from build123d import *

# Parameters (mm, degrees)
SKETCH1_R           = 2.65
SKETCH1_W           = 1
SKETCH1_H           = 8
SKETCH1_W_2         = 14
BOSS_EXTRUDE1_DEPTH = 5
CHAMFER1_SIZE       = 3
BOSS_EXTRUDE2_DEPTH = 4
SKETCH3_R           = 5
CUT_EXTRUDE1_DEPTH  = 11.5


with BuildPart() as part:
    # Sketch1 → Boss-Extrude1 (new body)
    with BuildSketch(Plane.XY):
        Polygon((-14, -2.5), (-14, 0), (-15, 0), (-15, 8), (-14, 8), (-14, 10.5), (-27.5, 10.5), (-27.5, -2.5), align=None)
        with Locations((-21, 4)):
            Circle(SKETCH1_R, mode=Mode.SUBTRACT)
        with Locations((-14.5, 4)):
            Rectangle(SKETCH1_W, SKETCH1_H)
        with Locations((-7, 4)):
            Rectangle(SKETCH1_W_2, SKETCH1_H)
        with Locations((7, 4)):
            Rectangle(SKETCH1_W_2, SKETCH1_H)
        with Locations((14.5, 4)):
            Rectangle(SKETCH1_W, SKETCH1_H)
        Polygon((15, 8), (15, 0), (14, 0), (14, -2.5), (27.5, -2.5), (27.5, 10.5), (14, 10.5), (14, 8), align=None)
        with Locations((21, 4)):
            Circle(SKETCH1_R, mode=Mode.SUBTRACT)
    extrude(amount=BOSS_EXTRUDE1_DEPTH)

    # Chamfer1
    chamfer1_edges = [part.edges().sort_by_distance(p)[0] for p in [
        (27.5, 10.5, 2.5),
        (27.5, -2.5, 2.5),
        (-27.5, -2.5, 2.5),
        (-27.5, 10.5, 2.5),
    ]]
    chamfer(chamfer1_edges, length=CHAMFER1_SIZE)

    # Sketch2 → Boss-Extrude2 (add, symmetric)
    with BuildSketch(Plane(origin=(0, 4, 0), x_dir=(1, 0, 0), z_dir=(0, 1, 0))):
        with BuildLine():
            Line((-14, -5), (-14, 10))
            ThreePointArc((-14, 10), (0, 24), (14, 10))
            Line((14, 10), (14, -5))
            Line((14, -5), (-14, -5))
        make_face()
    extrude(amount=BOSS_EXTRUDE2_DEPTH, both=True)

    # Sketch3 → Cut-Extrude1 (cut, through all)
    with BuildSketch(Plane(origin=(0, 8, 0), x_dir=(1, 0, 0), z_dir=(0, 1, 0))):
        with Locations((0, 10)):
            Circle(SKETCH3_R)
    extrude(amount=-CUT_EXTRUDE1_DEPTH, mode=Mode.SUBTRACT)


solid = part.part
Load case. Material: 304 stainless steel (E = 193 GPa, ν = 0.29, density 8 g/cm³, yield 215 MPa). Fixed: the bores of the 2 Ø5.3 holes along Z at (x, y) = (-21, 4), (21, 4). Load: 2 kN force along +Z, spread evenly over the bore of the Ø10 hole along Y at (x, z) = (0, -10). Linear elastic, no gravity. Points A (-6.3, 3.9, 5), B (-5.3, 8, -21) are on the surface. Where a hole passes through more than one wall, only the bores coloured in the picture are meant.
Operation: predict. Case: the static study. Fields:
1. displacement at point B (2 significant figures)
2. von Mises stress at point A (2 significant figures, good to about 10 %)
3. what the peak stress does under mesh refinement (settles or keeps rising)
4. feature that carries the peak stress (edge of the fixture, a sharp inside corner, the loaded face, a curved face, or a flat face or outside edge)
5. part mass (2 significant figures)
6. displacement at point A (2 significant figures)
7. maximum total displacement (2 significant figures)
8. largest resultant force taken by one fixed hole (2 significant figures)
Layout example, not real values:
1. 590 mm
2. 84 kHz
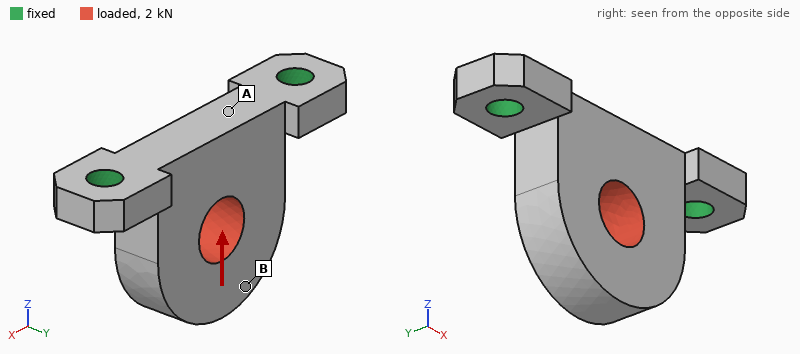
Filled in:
1. 5.5 µm
2. 18 MPa
3. keeps rising
4. edge of the fixture
5. 53 g
6. 5.4 µm
7. 6.1 µm
8. 1.1 kN
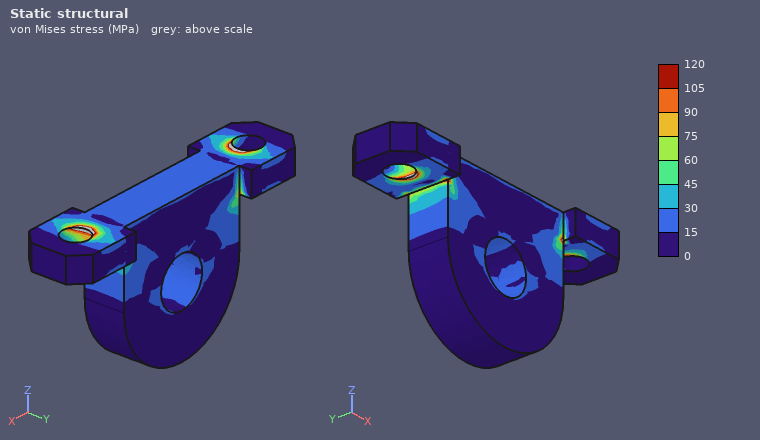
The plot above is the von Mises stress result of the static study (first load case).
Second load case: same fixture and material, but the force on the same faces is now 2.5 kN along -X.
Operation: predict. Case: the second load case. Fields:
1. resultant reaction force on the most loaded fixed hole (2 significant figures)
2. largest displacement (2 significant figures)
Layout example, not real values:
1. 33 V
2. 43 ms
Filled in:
1. 1.6 kN
2. 11 µm
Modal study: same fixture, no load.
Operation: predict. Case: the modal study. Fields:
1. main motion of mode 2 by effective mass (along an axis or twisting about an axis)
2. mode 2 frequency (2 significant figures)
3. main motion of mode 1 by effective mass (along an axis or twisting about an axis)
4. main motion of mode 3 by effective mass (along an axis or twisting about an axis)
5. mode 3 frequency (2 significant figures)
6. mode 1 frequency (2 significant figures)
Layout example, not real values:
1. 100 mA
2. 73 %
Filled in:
1. along X
2. 14 kHz
3. along Y
4. along Z
5. 15 kHz
6. 4400 Hz
